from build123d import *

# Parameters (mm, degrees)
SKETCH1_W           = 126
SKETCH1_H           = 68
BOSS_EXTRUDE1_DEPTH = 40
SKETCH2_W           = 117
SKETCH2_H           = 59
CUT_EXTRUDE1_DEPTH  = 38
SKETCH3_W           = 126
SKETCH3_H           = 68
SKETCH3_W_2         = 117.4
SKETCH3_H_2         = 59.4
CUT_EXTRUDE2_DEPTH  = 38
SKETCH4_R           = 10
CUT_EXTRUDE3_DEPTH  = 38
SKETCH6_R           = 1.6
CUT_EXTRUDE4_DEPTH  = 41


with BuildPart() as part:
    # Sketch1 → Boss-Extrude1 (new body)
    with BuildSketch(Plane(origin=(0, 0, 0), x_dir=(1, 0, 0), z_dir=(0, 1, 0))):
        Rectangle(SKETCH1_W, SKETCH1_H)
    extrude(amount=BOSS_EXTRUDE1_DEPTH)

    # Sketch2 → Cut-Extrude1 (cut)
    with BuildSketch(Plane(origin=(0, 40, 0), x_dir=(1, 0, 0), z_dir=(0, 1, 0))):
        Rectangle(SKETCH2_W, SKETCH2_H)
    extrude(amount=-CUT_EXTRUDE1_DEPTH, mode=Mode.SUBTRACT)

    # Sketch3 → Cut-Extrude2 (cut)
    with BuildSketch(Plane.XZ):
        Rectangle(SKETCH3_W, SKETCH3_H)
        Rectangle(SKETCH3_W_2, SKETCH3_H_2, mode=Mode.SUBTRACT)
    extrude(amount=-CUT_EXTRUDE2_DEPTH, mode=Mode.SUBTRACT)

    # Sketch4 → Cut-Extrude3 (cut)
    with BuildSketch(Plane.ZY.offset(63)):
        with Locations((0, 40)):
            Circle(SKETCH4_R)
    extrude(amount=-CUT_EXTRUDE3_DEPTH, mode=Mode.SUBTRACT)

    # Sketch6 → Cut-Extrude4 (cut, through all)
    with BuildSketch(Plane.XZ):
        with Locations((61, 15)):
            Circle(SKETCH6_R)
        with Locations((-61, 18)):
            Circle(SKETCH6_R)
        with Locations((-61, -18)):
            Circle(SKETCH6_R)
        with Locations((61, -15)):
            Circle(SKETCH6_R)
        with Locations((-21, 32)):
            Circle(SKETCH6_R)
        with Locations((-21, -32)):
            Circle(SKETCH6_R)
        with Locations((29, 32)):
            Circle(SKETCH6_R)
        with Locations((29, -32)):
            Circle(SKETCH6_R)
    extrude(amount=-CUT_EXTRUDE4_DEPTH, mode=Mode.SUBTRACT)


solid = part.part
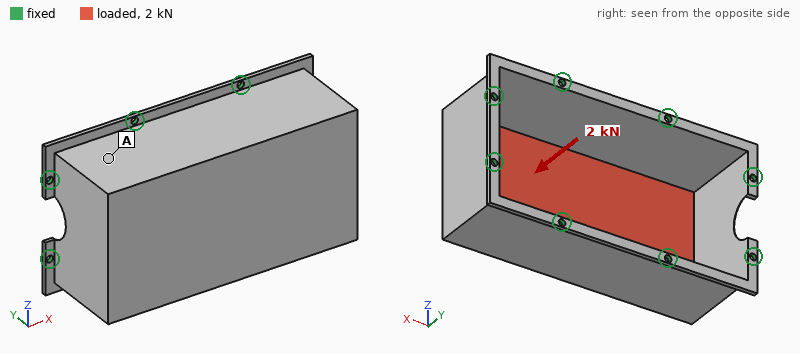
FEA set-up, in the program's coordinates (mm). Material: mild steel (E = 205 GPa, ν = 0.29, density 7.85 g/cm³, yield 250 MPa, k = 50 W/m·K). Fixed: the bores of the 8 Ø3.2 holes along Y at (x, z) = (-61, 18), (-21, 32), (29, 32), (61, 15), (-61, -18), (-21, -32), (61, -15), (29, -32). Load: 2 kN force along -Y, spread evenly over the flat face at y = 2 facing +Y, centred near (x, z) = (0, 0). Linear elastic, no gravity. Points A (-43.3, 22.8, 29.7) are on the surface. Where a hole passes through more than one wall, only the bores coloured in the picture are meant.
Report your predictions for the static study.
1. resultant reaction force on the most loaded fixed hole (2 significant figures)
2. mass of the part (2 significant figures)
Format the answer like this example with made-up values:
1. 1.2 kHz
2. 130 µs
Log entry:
1. 330 N
2. 150 g
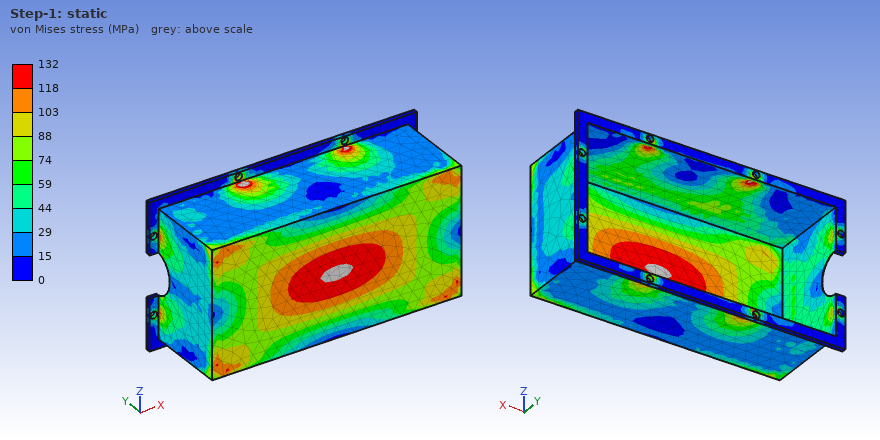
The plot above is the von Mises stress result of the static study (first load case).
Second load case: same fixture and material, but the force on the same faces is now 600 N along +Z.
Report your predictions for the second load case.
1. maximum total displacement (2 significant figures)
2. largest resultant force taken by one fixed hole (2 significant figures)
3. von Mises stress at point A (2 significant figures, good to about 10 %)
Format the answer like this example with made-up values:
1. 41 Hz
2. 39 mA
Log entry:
1. 28 µm
2. 210 N
3. 22 MPa
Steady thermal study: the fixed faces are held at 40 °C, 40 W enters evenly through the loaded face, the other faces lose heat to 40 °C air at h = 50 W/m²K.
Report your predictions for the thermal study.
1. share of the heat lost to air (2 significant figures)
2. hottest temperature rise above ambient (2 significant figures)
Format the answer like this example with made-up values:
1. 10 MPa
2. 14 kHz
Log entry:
1. 98 %
2. 65 K
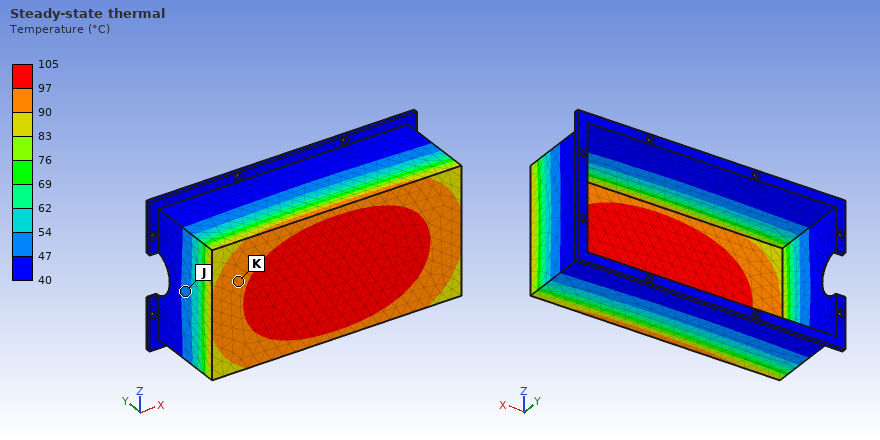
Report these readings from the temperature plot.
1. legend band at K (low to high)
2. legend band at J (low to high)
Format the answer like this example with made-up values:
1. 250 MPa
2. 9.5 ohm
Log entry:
1. 90 to 97 °C
2. 47 to 54 °C
